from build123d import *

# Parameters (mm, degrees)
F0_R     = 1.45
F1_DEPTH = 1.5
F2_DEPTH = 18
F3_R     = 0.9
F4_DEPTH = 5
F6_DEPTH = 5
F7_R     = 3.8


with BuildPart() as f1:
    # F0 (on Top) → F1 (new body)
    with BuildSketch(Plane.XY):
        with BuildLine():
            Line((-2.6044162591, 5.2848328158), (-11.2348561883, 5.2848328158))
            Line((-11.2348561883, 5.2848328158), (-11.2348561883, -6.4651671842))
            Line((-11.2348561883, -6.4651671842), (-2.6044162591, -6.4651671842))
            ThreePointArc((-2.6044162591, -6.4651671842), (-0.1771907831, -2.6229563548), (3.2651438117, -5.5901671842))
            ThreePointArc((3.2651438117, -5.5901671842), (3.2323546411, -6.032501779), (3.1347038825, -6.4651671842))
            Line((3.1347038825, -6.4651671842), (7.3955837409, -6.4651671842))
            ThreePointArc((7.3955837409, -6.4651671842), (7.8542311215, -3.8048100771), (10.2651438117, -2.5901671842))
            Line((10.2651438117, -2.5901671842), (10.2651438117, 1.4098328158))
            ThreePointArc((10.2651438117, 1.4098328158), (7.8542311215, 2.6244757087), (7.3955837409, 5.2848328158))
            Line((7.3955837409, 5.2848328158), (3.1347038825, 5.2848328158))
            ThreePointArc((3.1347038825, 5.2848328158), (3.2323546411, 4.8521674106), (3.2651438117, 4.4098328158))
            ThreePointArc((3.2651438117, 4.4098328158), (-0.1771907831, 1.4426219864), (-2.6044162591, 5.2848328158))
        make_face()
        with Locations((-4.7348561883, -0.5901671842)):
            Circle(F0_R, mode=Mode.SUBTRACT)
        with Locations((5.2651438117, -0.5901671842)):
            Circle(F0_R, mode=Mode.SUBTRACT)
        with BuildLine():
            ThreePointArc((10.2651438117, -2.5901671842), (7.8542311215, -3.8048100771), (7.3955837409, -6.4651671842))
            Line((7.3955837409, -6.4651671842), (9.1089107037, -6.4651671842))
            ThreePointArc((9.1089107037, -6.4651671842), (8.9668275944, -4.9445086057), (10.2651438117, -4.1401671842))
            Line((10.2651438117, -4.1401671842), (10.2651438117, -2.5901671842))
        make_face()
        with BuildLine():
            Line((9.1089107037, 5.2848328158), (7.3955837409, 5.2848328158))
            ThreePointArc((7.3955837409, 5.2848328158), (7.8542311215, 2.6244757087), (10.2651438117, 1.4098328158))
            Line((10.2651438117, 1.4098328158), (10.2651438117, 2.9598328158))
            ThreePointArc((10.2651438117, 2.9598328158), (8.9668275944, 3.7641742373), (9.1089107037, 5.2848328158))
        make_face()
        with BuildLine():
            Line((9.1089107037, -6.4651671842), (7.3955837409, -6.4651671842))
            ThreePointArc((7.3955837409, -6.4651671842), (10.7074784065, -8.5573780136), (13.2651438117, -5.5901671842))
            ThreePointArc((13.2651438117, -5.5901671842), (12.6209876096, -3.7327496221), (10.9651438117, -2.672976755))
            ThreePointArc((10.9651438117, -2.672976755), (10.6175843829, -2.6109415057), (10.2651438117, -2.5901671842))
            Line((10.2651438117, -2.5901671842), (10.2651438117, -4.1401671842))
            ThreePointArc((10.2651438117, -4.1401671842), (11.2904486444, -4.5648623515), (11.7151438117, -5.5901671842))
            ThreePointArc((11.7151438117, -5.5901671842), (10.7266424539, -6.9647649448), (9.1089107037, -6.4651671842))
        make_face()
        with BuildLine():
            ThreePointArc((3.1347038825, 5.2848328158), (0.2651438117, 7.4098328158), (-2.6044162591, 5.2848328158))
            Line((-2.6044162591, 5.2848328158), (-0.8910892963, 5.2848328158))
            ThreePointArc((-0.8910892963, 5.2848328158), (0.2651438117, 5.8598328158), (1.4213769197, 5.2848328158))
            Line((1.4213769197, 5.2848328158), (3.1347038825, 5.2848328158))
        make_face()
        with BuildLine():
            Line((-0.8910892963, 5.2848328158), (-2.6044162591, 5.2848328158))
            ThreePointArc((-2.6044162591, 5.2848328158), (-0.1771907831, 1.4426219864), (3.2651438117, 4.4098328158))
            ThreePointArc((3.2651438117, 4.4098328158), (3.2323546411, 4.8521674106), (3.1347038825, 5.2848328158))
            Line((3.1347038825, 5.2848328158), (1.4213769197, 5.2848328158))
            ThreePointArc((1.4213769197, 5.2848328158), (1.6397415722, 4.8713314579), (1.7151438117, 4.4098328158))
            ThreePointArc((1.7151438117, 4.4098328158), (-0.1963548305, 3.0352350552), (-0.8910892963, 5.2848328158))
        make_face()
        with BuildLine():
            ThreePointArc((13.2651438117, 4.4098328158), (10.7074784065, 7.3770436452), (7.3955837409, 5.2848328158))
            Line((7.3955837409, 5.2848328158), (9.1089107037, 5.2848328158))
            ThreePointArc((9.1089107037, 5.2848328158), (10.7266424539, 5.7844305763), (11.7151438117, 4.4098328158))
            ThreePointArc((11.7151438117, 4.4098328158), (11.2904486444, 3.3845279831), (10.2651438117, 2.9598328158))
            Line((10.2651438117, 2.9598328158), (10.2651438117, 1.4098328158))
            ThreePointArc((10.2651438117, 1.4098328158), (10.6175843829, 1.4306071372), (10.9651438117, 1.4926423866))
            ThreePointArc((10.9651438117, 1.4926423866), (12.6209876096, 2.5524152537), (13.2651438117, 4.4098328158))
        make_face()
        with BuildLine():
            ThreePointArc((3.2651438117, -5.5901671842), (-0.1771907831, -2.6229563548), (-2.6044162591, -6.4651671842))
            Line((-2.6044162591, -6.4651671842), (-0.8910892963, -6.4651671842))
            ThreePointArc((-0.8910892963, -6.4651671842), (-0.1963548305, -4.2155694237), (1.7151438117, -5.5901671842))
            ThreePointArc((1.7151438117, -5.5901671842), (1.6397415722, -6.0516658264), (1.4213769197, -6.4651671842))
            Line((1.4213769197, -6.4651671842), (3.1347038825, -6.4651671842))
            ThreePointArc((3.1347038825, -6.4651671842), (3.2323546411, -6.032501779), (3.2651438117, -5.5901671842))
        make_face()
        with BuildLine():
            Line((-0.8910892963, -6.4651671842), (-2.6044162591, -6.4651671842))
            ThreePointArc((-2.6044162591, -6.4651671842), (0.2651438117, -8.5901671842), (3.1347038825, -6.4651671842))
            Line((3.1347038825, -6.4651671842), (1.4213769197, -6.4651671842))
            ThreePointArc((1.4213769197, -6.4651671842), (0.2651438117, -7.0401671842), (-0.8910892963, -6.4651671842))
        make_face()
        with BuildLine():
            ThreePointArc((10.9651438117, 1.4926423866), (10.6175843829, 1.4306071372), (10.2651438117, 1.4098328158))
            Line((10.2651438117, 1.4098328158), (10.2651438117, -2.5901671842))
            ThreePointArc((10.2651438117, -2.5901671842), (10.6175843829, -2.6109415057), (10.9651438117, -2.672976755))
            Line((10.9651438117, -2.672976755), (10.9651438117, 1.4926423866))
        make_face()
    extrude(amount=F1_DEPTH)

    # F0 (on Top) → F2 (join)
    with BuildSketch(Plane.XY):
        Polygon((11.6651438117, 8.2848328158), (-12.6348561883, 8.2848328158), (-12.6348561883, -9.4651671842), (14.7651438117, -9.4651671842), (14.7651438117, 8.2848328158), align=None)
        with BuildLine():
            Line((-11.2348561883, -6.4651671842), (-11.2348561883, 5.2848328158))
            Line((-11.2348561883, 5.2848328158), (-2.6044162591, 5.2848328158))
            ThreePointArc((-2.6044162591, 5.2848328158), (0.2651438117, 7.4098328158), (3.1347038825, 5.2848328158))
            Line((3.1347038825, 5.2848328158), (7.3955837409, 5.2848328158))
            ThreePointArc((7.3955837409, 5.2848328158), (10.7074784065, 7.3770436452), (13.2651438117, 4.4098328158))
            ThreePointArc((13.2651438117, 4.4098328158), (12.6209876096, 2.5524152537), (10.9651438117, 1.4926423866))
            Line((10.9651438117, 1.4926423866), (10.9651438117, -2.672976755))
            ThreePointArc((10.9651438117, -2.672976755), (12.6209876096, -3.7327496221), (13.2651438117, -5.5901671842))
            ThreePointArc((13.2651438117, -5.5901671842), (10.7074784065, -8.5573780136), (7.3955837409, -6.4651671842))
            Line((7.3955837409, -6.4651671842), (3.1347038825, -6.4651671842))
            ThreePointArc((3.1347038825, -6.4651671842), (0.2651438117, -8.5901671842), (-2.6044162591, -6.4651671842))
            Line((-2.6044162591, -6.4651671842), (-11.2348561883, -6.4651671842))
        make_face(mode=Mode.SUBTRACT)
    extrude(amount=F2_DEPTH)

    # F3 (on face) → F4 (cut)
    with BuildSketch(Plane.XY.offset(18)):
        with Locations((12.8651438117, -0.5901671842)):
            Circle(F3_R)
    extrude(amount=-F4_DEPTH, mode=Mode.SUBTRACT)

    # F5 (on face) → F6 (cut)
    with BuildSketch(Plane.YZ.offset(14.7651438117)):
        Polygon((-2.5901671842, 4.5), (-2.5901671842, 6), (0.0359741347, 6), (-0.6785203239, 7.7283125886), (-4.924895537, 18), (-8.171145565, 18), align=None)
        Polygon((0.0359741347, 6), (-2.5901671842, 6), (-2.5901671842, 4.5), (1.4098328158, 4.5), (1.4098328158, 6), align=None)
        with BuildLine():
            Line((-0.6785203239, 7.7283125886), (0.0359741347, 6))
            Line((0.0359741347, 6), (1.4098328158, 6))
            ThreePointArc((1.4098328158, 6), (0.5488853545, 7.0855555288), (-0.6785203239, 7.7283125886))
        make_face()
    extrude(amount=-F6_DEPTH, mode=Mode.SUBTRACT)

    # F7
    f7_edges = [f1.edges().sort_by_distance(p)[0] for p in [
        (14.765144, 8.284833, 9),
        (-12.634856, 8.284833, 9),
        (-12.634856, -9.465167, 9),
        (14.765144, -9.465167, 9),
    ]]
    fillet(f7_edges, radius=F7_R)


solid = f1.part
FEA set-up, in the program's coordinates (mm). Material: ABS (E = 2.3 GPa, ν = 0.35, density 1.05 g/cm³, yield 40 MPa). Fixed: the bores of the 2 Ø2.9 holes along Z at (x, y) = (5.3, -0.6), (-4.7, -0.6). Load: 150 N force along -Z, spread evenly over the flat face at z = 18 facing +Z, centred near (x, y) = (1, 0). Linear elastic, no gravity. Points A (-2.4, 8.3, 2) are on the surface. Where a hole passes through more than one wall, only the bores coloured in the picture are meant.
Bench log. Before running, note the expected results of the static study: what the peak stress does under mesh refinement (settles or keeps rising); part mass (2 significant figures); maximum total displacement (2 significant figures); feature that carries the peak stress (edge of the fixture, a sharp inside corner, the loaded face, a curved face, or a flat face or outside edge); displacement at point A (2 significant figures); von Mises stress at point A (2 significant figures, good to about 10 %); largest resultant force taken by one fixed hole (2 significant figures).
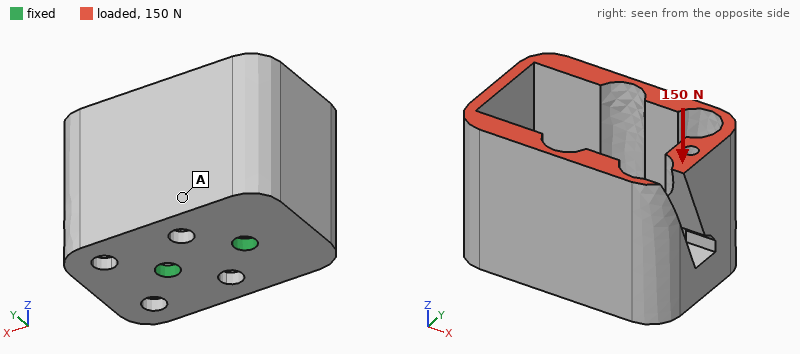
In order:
keeps rising
3.4 g
0.20 mm
edge of the fixture
0.15 mm
4.1 MPa
78 N
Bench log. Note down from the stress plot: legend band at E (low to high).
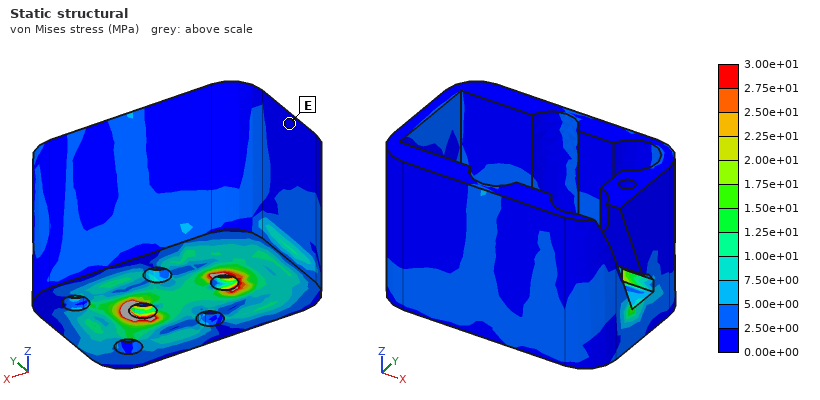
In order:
0.00e+00 to 2.50e+00 MPa
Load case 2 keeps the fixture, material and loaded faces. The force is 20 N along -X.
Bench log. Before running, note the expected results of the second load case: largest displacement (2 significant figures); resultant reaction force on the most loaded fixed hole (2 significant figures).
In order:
0.36 mm
27 N
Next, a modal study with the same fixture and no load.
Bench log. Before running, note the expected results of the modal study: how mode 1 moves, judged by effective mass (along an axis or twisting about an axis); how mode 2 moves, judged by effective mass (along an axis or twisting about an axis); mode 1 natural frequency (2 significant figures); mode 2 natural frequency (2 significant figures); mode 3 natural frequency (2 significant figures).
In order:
along Y
along X
910 Hz
1400 Hz
1900 Hz
